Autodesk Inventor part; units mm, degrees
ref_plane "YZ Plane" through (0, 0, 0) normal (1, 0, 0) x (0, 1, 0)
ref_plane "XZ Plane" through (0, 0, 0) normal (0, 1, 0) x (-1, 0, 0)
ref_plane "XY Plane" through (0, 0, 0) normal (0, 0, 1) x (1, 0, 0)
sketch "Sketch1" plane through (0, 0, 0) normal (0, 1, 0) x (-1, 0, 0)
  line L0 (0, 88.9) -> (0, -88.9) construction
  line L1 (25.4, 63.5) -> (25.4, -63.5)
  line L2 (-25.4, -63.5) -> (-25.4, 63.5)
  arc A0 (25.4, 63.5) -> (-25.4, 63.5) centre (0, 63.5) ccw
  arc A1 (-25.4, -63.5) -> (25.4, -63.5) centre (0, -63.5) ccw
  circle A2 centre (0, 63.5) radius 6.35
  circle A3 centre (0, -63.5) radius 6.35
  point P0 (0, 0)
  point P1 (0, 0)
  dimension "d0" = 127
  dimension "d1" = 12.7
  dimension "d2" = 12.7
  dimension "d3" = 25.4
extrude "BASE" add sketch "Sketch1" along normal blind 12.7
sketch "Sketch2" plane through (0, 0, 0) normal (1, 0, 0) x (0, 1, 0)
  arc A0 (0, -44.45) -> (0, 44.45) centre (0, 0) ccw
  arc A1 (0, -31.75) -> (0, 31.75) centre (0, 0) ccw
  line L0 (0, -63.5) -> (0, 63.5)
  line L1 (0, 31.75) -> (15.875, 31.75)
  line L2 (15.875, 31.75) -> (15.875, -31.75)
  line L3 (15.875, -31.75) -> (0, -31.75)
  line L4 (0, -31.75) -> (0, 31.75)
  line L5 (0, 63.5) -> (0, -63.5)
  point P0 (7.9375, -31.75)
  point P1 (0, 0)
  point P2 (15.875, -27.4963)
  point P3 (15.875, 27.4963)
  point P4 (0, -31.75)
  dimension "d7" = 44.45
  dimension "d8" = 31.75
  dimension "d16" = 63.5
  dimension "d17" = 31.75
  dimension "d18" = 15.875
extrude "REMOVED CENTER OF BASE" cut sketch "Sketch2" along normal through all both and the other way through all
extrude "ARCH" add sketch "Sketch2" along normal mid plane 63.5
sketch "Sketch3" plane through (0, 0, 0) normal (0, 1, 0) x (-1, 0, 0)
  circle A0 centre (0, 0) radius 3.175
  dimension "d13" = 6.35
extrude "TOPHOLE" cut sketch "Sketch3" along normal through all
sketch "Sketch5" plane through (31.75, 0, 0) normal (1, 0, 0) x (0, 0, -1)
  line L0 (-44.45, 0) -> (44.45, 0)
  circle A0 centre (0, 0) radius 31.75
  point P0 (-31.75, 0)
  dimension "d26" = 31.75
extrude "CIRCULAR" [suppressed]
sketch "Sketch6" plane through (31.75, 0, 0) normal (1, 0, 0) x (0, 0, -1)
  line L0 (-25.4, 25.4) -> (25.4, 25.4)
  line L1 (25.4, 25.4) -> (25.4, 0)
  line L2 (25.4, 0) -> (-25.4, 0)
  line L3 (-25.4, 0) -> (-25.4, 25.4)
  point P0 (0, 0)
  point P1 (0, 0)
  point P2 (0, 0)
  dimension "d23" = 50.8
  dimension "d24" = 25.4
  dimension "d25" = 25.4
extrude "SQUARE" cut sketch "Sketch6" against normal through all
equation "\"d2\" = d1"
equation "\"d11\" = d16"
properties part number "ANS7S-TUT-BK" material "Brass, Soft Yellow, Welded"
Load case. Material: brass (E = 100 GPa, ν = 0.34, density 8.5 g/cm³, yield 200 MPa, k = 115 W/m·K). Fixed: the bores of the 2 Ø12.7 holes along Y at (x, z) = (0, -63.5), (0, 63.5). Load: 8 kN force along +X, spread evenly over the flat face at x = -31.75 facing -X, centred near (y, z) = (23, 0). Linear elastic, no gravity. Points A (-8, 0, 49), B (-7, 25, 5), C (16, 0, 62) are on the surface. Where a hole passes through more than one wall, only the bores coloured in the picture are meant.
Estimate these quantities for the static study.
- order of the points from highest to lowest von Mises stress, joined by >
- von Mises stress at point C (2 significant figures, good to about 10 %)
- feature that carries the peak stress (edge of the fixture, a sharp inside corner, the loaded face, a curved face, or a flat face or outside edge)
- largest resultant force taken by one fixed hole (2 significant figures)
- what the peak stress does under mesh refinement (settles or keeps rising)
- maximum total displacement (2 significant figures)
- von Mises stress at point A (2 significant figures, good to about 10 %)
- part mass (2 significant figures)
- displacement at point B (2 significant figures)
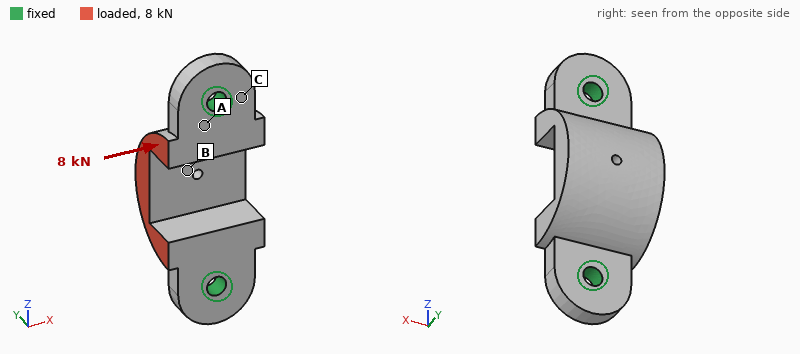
C > A > B
30 MPa
edge of the fixture
4.0 kN
keeps rising
84 µm
17 MPa
1.4 kg
44 µm
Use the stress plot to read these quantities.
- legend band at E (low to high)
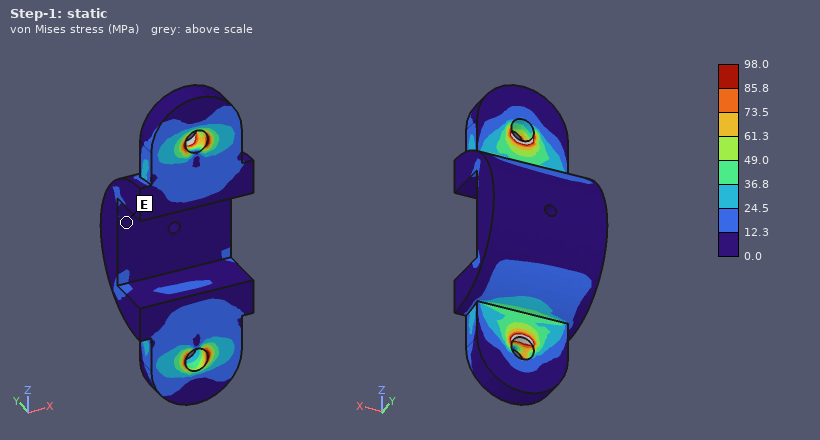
0.0 to 12.3 MPa
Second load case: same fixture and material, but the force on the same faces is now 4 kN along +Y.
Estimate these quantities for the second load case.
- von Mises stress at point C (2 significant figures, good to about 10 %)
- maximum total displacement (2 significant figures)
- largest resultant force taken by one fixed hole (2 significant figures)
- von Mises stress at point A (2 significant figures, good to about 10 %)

18 MPa
66 µm
2.6 kN
27 MPa
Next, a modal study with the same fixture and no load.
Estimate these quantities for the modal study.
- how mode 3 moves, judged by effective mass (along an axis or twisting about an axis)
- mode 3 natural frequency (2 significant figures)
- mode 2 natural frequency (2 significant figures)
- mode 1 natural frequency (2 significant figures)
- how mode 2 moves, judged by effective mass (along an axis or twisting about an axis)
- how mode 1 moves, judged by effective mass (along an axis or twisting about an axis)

along Z
3800 Hz
3600 Hz
1800 Hz
along Y
along X
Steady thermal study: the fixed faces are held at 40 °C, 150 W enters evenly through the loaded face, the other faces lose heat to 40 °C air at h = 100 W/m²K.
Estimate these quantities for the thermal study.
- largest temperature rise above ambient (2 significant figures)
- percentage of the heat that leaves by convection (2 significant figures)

45 K
33 %
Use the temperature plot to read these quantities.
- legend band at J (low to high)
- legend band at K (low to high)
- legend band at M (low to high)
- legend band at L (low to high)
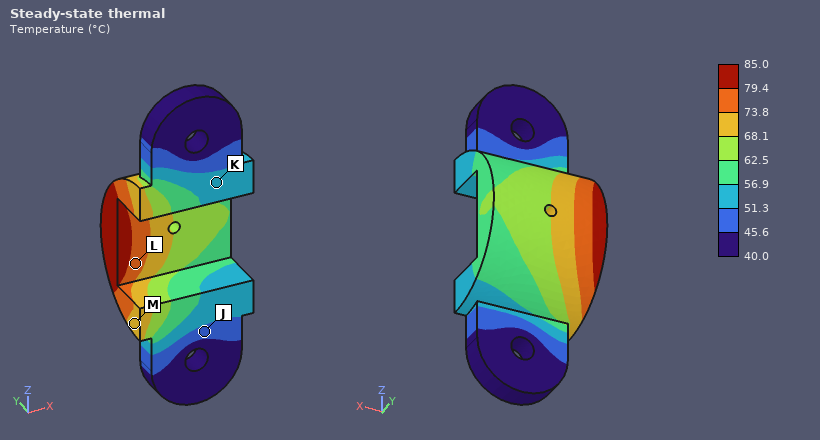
45.6 to 51.3 °C
51.3 to 56.9 °C
68.1 to 73.8 °C
73.8 to 79.4 °C
